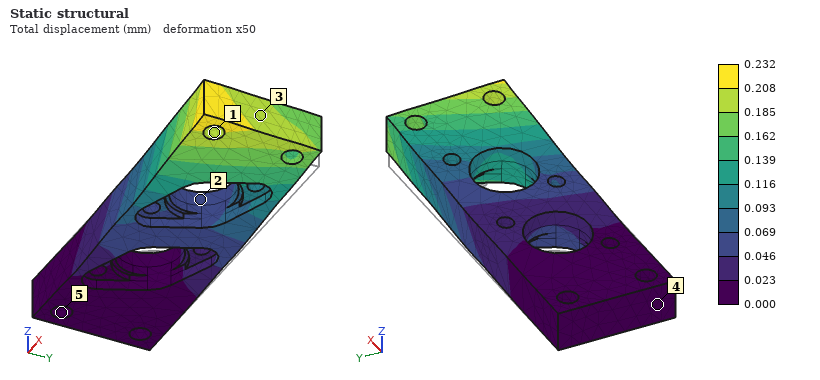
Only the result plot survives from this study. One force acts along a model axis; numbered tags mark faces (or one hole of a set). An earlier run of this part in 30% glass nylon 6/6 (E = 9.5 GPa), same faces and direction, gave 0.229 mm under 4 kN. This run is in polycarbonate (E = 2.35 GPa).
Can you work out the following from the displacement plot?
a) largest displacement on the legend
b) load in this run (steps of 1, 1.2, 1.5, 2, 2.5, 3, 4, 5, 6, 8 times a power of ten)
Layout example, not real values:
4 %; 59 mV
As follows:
0.232 mm; 1 kN
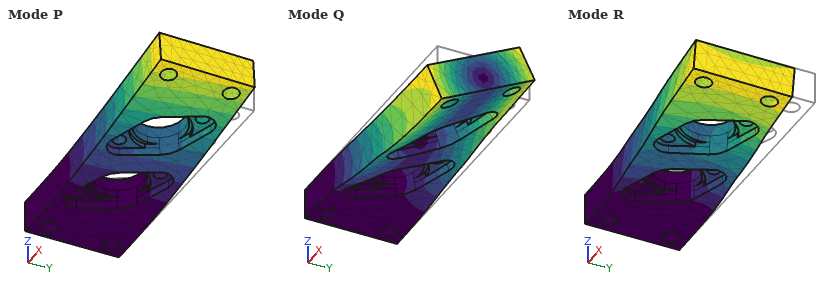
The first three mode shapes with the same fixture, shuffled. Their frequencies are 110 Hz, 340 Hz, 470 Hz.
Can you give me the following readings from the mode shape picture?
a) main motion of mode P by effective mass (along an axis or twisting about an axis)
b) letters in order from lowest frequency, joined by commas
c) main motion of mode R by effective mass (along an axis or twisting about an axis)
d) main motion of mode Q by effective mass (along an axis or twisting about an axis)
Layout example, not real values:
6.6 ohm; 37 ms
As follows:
along Z; P, R, Q; along Y; twisting about X
